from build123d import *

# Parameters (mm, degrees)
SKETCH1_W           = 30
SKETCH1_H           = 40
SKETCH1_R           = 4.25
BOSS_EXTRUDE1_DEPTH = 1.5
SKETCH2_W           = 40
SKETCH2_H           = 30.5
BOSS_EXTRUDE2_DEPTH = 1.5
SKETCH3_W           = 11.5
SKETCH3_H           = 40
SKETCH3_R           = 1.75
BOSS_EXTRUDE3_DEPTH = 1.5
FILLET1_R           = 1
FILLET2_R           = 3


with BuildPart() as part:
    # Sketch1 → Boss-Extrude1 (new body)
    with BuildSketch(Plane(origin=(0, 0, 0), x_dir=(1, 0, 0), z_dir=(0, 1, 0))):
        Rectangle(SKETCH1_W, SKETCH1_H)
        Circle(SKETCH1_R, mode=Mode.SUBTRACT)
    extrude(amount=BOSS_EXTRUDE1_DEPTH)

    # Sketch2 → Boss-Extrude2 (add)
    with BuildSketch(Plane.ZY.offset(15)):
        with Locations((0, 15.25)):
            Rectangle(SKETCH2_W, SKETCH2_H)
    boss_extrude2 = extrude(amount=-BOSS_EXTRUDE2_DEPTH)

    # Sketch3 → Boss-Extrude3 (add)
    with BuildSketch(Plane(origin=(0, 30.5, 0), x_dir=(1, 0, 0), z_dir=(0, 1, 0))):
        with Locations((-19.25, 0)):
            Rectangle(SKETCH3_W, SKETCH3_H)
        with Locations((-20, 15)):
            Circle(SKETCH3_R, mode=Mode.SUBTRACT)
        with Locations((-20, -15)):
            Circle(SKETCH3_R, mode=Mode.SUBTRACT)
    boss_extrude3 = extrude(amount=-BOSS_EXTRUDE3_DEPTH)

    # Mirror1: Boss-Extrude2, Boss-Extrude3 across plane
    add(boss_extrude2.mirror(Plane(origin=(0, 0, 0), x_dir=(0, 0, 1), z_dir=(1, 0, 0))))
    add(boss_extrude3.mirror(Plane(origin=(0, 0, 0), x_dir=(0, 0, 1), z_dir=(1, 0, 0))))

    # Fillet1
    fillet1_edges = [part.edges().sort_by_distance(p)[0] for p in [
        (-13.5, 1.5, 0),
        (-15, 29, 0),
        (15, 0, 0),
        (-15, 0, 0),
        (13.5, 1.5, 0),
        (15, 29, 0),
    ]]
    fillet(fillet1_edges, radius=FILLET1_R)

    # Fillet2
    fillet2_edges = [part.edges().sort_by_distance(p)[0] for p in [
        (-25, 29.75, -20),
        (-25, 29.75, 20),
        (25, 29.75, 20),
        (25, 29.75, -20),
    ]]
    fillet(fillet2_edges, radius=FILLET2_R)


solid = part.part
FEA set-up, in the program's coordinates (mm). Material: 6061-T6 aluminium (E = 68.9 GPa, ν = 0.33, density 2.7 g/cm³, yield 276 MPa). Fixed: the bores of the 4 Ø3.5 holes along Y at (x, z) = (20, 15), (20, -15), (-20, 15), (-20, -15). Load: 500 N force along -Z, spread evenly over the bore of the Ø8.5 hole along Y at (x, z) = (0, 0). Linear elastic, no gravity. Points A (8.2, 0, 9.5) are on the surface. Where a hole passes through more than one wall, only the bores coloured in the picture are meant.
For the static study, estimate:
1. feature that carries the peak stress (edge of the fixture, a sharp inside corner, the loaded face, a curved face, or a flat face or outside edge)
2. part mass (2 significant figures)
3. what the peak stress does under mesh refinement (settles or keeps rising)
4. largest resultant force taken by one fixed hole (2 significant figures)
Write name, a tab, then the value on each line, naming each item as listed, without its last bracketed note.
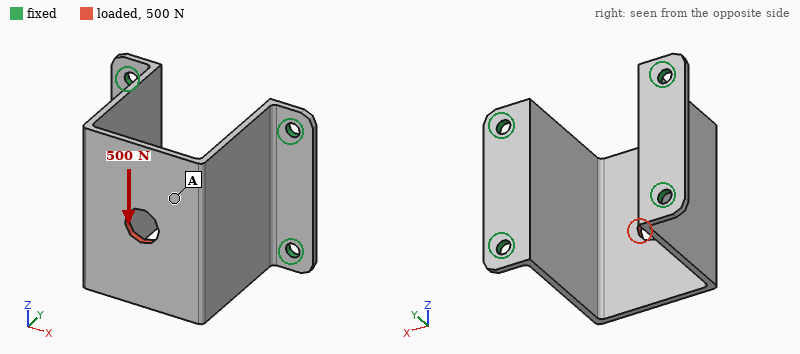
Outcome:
feature that carries the peak stress	edge of the fixture
part mass	17 g
what the peak stress does under mesh refinement	keeps rising
largest resultant force taken by one fixed hole	270 N
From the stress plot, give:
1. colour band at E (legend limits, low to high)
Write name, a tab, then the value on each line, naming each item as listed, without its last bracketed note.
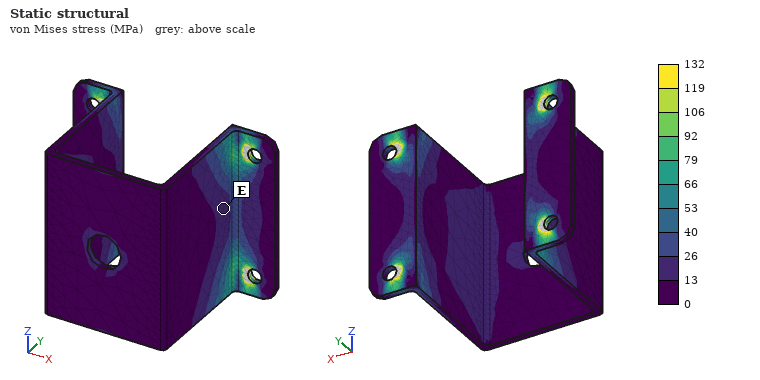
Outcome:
colour band at E	13 to 26 MPa
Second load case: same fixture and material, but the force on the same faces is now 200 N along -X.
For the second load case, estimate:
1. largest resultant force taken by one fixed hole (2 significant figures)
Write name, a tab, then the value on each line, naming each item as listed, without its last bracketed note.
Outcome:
largest resultant force taken by one fixed hole	75 N
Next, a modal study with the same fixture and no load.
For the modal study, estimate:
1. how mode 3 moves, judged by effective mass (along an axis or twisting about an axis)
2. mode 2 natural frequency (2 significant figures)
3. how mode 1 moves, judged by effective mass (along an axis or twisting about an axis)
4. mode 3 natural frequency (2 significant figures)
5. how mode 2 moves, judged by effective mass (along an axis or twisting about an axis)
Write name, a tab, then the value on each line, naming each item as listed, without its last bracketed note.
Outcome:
how mode 3 moves, judged by effective mass	along Z
mode 2 natural frequency	3800 Hz
how mode 1 moves, judged by effective mass	along X
mode 3 natural frequency	4700 Hz
how mode 2 moves, judged by effective mass	twisting about Y
